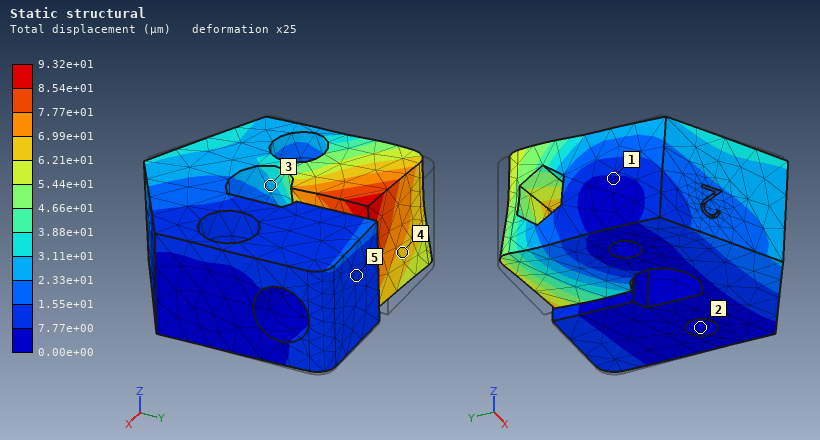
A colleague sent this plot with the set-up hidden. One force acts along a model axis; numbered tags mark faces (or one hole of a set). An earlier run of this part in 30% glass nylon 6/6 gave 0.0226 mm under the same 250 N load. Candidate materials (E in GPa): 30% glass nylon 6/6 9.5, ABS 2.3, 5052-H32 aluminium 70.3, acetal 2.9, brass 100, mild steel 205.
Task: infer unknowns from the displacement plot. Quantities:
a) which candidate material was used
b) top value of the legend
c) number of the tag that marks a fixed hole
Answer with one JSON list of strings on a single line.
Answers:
["ABS", "9.32e+01 µm", "2"]
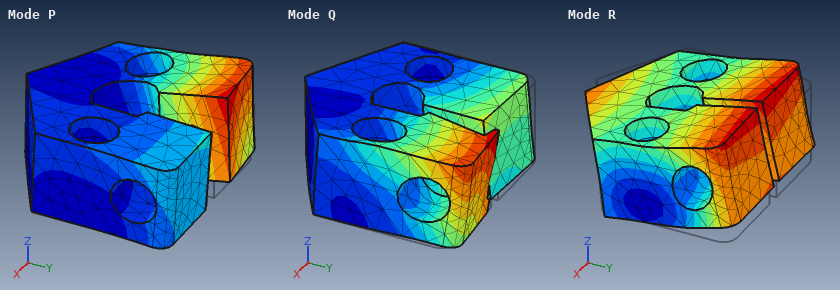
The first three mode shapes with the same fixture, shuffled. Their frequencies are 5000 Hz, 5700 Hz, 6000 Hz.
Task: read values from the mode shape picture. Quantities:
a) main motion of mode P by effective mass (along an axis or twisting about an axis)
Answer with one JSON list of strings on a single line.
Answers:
["along X"]
